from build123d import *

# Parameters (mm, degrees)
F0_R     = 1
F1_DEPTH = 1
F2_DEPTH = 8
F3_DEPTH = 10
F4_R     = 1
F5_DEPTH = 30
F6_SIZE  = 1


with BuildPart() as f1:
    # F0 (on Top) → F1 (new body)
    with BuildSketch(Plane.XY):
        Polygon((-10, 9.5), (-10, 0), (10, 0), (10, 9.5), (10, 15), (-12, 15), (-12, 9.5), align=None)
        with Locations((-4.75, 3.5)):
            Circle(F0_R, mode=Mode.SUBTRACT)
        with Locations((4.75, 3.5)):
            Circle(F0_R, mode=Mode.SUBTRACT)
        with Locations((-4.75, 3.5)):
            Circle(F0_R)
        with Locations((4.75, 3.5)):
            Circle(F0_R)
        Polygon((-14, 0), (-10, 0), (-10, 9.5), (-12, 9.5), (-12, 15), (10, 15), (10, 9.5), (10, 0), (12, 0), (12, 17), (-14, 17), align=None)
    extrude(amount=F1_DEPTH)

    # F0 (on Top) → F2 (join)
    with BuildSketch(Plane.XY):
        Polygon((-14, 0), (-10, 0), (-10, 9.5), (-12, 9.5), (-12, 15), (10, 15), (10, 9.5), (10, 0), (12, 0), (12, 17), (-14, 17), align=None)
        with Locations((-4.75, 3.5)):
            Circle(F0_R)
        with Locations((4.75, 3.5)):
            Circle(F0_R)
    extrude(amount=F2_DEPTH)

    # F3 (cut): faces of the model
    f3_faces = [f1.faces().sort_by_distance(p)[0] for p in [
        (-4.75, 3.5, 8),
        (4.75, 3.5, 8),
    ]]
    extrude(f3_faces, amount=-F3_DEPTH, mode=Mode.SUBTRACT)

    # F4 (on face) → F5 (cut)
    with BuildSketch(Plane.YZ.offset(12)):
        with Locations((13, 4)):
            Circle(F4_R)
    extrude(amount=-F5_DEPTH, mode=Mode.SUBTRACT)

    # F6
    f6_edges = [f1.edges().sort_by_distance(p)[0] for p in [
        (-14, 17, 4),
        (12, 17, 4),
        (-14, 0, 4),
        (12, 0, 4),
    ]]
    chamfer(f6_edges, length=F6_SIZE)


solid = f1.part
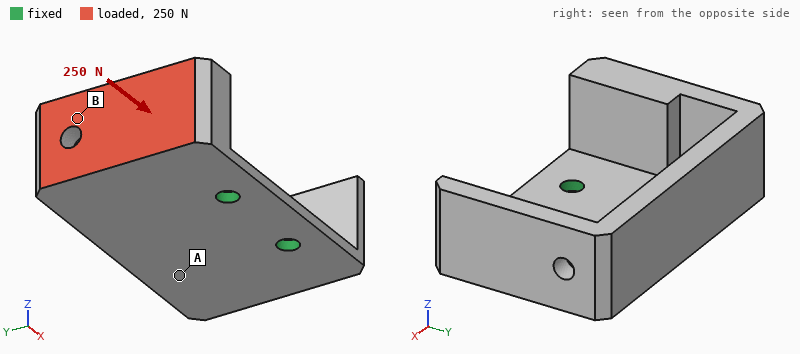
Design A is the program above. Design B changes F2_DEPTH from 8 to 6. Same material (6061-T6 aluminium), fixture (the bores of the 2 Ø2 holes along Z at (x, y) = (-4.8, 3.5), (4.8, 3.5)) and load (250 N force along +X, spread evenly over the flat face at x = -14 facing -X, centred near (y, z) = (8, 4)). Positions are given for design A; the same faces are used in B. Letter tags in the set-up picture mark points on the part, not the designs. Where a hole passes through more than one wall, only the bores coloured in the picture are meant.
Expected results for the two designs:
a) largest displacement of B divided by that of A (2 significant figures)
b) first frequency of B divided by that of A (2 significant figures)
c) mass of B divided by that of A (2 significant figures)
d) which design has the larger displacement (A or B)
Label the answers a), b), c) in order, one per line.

a) 0.75
b) 1.2
c) 0.81
d) A
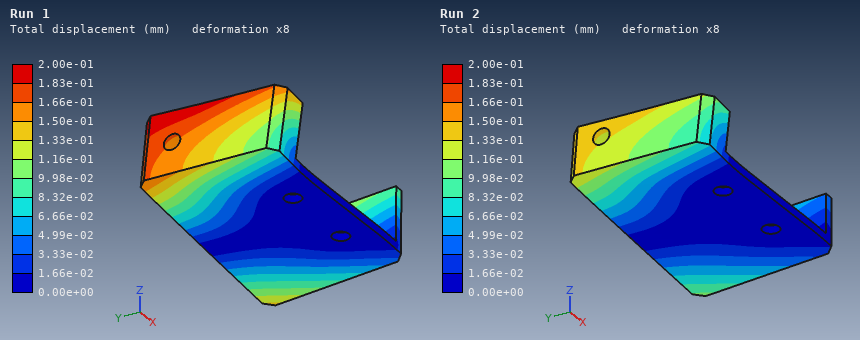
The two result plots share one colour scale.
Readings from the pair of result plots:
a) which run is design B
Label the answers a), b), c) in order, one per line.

a) Run 2
